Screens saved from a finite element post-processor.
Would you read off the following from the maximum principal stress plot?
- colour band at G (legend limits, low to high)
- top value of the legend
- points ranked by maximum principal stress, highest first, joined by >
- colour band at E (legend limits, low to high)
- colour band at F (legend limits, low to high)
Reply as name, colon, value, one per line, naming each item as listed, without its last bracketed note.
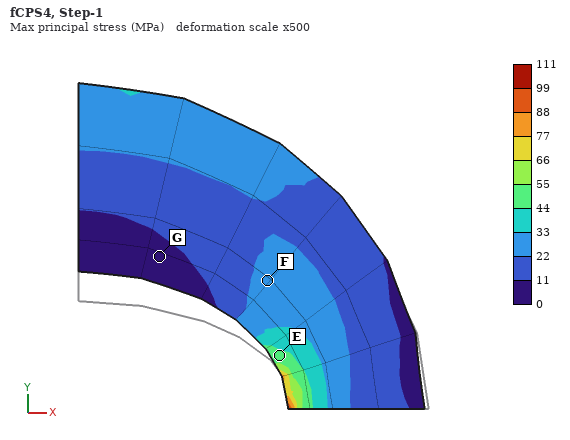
colour band at G: 0 to 11 MPa
top value of the legend: 111 MPa
points ranked by maximum principal stress, highest first, joined by >: E > F > G
colour band at E: 44 to 55 MPa
colour band at F: 22 to 33 MPa
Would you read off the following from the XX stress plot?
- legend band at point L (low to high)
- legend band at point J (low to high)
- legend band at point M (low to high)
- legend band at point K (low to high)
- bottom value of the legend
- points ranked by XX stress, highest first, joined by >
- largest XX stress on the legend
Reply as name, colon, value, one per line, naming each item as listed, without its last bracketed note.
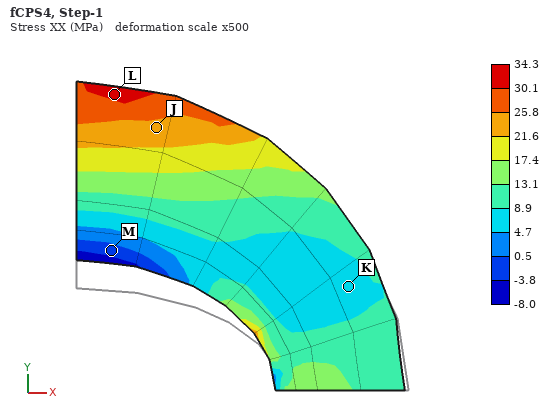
legend band at point L: 30.1 to 34.3 MPa
legend band at point J: 21.6 to 25.8 MPa
legend band at point M: -3.8 to 0.5 MPa
legend band at point K: 4.7 to 8.9 MPa
bottom value of the legend: -8.0 MPa
points ranked by XX stress, highest first, joined by >: L > J > K > M
largest XX stress on the legend: 34.3 MPa
